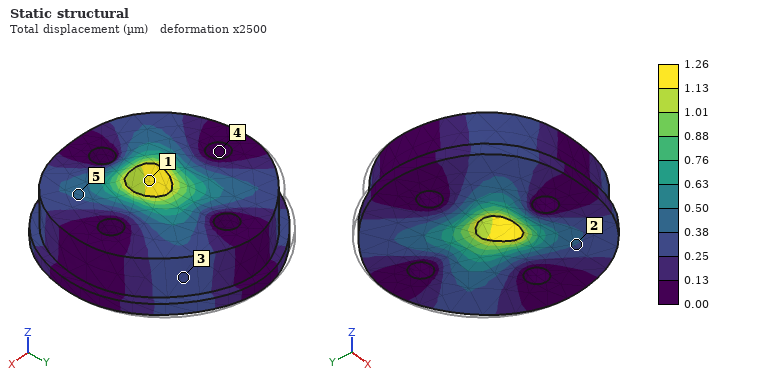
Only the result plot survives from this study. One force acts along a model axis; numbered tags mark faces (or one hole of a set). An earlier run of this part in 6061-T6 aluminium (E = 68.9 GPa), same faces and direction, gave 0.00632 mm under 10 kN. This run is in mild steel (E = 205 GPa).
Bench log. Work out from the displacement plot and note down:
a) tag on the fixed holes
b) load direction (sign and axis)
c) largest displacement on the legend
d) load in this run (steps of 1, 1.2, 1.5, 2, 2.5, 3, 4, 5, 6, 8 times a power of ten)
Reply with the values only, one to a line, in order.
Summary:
4
-Y
1.26 µm
6 kN
